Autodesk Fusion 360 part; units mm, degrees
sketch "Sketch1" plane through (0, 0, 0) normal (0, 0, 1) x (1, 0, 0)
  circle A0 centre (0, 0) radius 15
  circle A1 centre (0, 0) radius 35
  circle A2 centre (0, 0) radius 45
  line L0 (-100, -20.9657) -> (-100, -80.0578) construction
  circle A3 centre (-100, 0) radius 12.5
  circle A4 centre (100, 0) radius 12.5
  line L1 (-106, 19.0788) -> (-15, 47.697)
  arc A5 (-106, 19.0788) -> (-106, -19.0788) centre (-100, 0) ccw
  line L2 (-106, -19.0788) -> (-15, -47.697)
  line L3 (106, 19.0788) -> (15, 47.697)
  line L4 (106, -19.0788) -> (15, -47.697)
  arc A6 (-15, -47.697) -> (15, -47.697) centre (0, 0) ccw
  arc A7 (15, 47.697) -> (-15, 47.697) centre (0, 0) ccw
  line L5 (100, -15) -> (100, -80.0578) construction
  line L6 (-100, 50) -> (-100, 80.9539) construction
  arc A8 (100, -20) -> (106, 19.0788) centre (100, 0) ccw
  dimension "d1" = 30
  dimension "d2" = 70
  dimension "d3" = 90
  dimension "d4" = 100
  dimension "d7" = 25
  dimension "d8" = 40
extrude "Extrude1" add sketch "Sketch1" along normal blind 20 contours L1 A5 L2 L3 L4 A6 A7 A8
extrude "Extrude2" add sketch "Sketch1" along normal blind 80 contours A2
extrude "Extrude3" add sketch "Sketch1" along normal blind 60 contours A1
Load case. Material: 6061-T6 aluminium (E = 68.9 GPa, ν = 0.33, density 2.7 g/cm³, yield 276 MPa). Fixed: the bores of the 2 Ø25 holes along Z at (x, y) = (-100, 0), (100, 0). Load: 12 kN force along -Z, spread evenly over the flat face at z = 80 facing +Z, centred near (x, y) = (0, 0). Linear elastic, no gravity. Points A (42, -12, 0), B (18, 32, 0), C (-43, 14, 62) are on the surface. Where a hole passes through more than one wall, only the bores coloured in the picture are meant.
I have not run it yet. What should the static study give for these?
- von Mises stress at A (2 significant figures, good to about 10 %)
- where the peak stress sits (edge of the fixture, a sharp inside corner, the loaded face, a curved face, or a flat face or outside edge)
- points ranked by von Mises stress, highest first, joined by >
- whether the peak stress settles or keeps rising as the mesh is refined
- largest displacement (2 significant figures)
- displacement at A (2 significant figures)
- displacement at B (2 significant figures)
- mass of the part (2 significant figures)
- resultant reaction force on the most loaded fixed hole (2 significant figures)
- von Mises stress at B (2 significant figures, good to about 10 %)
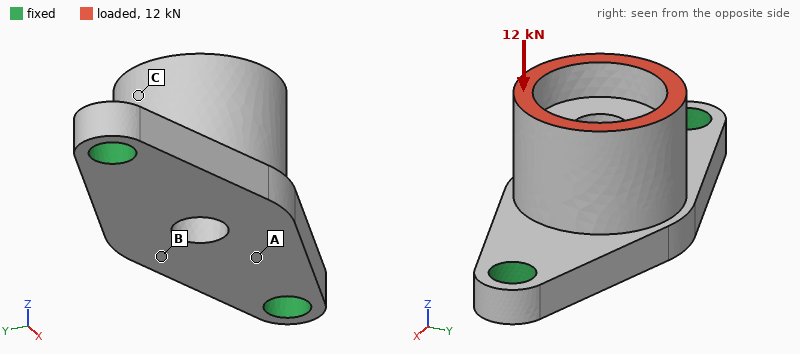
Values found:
19 MPa
edge of the fixture
A > B > C
keeps rising
60 µm
48 µm
55 µm
1.5 kg
6.6 kN
9.7 MPa
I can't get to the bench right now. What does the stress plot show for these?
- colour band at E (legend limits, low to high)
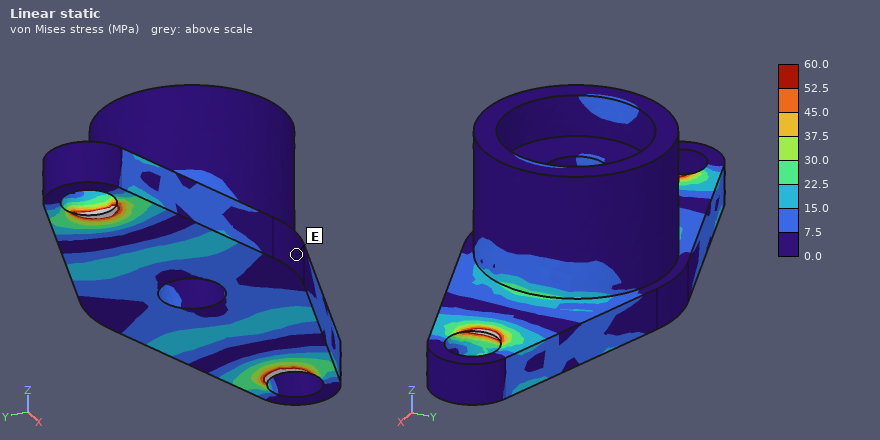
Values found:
0.0 to 7.5 MPa
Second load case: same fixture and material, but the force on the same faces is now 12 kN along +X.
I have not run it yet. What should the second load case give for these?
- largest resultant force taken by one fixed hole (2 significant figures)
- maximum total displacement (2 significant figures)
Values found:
8.4 kN
91 µm
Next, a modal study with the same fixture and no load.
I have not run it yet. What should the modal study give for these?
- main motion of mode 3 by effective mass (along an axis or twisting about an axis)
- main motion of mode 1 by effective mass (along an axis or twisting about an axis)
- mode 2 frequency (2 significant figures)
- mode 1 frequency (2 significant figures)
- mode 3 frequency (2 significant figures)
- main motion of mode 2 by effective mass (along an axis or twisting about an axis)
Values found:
along X
along Y
2100 Hz
1300 Hz
3600 Hz
along Z
